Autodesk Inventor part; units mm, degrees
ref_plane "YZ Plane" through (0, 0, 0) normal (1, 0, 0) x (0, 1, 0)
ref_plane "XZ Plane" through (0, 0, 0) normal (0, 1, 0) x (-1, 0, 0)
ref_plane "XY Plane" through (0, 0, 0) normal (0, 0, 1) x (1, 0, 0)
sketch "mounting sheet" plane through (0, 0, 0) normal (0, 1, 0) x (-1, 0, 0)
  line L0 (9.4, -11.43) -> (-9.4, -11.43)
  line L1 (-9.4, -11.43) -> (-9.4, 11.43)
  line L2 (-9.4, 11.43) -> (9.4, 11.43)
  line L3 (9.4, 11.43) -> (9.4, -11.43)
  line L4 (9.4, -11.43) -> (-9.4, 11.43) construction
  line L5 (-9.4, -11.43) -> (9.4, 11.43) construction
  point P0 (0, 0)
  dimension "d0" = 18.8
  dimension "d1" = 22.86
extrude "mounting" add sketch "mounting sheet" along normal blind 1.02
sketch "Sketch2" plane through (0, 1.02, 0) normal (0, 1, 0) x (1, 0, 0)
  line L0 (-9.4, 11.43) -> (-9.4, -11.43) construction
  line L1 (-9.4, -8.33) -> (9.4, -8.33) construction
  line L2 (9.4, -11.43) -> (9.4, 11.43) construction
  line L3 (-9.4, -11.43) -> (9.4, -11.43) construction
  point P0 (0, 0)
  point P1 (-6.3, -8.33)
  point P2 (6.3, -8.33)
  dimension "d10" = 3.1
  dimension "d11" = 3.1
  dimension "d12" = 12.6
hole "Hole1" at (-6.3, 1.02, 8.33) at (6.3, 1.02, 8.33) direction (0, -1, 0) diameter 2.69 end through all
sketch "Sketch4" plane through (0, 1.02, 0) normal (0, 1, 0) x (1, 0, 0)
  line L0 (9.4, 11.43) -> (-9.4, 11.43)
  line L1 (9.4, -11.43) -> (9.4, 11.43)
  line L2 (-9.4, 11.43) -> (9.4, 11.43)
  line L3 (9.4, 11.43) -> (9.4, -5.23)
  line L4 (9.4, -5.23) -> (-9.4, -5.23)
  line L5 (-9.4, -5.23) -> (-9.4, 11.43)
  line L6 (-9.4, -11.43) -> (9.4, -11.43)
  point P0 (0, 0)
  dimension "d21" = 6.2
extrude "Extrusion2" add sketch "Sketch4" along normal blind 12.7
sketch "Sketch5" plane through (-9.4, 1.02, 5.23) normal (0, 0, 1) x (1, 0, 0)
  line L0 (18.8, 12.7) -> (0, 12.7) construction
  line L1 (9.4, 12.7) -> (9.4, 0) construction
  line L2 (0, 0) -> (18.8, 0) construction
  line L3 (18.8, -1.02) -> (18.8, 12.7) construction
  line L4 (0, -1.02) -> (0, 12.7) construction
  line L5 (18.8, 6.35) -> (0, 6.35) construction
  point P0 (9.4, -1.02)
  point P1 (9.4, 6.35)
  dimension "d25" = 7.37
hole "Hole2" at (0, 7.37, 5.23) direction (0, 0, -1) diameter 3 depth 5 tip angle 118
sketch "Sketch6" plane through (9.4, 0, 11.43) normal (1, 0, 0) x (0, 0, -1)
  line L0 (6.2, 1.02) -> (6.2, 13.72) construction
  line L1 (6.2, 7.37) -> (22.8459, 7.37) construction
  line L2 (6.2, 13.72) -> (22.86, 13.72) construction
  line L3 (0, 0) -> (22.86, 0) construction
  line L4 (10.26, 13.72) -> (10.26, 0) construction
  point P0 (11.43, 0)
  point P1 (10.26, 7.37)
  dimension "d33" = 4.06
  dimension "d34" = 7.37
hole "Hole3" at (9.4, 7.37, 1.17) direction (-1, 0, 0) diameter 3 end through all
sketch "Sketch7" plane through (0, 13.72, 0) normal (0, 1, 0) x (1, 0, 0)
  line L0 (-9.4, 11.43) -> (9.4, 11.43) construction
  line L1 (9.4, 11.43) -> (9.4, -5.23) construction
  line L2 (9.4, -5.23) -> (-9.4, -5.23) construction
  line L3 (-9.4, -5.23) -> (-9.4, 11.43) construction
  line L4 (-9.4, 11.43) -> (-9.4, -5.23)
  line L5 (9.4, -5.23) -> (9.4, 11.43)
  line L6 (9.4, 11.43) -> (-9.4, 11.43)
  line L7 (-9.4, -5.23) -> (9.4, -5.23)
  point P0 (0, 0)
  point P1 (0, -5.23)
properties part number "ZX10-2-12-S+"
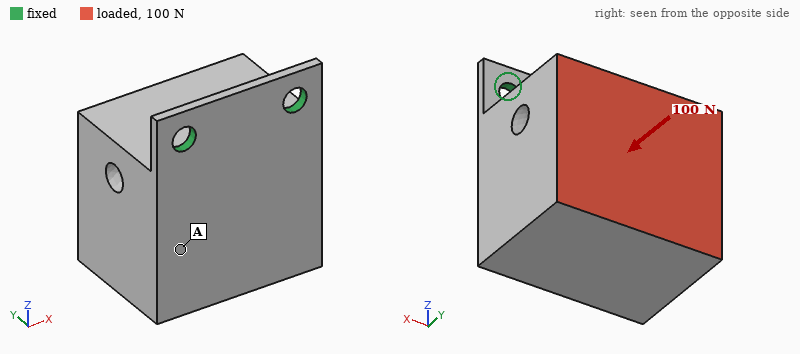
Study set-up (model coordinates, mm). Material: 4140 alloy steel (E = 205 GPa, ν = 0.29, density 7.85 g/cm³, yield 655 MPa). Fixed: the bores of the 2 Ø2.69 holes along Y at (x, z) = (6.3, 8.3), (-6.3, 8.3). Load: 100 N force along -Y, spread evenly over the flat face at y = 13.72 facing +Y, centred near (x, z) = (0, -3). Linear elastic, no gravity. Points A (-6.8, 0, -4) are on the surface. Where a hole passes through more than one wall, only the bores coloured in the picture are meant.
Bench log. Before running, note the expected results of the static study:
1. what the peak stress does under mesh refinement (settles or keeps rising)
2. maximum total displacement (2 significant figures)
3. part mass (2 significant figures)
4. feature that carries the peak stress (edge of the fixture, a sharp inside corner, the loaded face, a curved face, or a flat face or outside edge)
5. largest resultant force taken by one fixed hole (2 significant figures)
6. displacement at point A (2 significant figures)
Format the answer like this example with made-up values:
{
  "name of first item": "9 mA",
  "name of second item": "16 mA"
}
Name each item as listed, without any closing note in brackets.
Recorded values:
{
  "what the peak stress does under mesh refinement": "keeps rising",
  "maximum total displacement": "0.17 mm",
  "part mass": "33 g",
  "feature that carries the peak stress": "edge of the fixture",
  "largest resultant force taken by one fixed hole": "50 N",
  "displacement at point A": "0.079 mm"
}
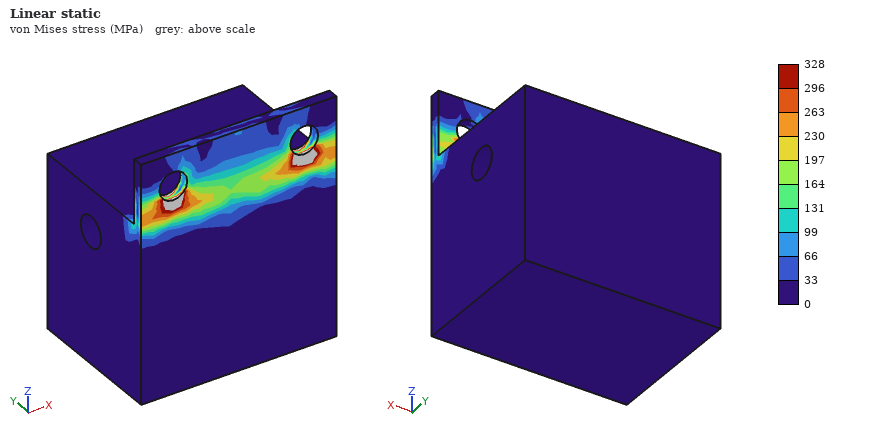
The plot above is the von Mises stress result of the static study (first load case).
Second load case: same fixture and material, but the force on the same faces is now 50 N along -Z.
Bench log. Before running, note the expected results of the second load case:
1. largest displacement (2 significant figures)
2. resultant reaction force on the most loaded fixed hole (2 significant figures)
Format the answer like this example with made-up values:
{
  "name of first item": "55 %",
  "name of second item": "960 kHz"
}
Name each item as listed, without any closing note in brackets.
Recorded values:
{
  "largest displacement": "0.12 mm",
  "resultant reaction force on the most loaded fixed hole": "25 N"
}
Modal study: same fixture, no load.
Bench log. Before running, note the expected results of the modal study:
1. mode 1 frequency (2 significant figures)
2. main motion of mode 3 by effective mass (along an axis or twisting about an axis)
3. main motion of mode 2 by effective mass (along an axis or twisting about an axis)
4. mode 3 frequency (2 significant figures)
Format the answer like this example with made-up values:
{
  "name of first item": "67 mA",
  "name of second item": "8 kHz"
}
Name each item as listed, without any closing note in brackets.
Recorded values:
{
  "mode 1 frequency": "750 Hz",
  "main motion of mode 3 by effective mass": "along X",
  "main motion of mode 2 by effective mass": "along X",
  "mode 3 frequency": "11 kHz"
}
